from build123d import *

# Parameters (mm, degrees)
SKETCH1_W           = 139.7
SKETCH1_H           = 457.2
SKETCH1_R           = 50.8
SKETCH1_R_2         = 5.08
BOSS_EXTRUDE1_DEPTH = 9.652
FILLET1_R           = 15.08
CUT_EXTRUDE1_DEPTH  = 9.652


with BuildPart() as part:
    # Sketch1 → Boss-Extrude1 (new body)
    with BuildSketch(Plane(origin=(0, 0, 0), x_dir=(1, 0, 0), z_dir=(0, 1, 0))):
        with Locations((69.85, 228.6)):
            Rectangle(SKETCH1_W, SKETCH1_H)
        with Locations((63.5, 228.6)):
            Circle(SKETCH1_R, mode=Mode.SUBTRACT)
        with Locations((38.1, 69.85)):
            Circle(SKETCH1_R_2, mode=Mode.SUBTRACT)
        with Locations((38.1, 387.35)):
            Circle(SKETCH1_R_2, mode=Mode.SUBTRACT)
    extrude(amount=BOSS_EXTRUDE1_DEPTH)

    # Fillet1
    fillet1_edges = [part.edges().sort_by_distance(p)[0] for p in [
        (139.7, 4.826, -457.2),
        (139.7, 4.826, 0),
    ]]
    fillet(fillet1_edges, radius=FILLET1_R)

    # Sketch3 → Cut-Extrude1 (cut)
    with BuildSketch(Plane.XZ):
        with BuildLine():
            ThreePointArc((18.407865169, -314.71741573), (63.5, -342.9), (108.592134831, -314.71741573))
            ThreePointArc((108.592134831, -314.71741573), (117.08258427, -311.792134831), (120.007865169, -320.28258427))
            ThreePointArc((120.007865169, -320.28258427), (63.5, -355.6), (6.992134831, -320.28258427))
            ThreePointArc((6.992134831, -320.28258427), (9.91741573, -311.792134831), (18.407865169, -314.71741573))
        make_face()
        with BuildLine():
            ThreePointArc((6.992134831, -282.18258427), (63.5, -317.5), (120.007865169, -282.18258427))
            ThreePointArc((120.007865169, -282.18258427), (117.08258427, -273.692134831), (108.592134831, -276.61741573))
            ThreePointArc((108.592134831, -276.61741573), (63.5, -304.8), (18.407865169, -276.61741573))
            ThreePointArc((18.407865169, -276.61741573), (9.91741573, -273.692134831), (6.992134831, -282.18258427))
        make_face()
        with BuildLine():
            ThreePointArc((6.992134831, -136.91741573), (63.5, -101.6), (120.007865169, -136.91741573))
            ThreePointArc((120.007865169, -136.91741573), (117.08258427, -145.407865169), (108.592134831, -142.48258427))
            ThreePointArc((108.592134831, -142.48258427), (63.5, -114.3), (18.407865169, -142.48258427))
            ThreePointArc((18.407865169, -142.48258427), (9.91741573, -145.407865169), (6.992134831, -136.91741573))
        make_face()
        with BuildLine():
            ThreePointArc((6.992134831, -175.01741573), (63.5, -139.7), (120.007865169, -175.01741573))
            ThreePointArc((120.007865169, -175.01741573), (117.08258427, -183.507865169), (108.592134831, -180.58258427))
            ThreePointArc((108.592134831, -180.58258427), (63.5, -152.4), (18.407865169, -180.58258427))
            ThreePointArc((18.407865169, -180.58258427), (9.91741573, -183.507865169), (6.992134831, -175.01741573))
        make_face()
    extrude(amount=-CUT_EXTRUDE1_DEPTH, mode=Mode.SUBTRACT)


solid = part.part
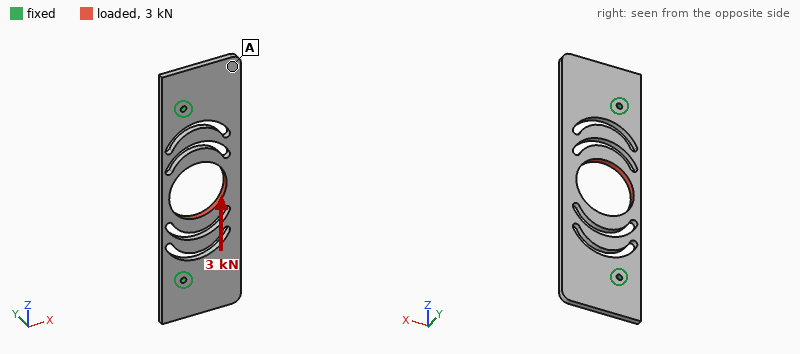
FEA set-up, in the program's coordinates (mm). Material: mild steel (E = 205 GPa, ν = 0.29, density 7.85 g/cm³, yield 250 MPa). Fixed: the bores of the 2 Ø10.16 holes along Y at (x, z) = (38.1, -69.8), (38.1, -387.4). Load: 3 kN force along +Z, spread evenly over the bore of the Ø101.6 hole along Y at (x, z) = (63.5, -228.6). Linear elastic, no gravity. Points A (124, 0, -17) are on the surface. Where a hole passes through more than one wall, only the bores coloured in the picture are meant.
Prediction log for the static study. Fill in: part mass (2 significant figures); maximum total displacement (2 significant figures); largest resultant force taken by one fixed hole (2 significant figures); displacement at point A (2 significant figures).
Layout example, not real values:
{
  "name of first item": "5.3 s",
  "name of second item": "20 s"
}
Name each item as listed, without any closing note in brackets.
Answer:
{
  "part mass": "3.7 kg",
  "maximum total displacement": "12 µm",
  "largest resultant force taken by one fixed hole": "1.5 kN",
  "displacement at point A": "8.9 µm"
}
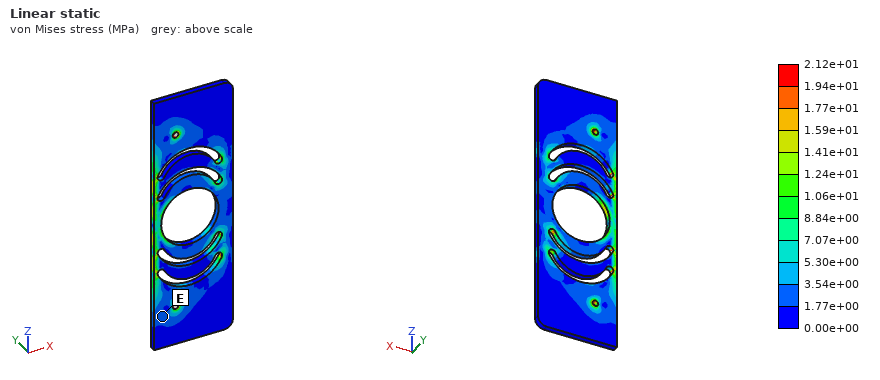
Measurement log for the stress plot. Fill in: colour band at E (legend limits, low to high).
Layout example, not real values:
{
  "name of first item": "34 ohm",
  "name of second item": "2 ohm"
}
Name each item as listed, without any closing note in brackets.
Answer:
{
  "colour band at E": "1.77e+00 to 3.54e+00 MPa"
}
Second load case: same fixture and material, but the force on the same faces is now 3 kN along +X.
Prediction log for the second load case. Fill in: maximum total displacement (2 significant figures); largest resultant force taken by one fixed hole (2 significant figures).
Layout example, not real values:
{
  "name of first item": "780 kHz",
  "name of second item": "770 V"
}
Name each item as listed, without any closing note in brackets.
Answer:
{
  "maximum total displacement": "51 µm",
  "largest resultant force taken by one fixed hole": "1.8 kN"
}
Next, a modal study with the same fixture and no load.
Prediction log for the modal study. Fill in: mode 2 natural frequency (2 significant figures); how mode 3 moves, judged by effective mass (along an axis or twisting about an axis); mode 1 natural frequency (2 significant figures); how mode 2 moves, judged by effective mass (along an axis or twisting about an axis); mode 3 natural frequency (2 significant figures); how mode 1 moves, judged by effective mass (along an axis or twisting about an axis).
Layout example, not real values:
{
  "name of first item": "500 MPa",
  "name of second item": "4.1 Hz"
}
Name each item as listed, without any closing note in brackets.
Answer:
{
  "mode 2 natural frequency": "550 Hz",
  "how mode 3 moves, judged by effective mass": "twisting about X",
  "mode 1 natural frequency": "340 Hz",
  "how mode 2 moves, judged by effective mass": "twisting about Z",
  "mode 3 natural frequency": "590 Hz",
  "how mode 1 moves, judged by effective mass": "along Y"
}
